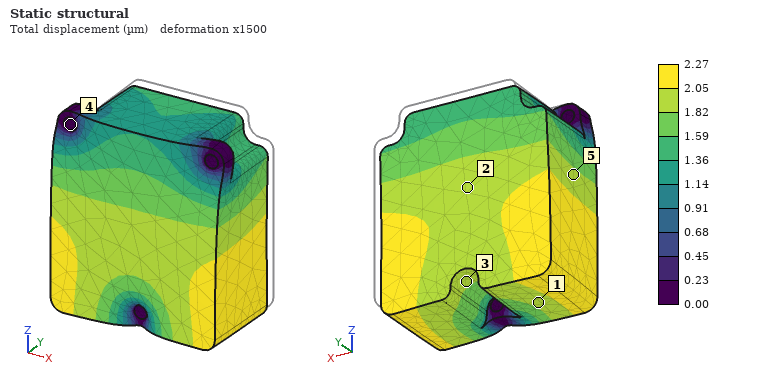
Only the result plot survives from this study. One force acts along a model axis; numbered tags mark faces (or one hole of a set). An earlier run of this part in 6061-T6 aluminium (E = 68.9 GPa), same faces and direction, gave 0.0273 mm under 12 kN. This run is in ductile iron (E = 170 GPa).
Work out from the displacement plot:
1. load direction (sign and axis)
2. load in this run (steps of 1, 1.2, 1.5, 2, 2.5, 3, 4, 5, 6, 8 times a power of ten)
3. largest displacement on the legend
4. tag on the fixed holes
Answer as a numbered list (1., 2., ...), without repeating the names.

1. -Y
2. 2.5 kN
3. 2.27 µm
4. 4
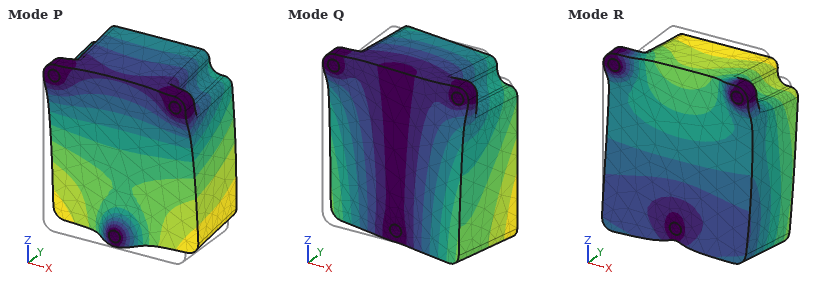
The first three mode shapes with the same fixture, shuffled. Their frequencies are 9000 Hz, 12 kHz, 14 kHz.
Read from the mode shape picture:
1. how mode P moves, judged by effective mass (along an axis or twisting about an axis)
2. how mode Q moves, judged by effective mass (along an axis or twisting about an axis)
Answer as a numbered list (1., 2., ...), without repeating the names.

1. along Y
2. along X
